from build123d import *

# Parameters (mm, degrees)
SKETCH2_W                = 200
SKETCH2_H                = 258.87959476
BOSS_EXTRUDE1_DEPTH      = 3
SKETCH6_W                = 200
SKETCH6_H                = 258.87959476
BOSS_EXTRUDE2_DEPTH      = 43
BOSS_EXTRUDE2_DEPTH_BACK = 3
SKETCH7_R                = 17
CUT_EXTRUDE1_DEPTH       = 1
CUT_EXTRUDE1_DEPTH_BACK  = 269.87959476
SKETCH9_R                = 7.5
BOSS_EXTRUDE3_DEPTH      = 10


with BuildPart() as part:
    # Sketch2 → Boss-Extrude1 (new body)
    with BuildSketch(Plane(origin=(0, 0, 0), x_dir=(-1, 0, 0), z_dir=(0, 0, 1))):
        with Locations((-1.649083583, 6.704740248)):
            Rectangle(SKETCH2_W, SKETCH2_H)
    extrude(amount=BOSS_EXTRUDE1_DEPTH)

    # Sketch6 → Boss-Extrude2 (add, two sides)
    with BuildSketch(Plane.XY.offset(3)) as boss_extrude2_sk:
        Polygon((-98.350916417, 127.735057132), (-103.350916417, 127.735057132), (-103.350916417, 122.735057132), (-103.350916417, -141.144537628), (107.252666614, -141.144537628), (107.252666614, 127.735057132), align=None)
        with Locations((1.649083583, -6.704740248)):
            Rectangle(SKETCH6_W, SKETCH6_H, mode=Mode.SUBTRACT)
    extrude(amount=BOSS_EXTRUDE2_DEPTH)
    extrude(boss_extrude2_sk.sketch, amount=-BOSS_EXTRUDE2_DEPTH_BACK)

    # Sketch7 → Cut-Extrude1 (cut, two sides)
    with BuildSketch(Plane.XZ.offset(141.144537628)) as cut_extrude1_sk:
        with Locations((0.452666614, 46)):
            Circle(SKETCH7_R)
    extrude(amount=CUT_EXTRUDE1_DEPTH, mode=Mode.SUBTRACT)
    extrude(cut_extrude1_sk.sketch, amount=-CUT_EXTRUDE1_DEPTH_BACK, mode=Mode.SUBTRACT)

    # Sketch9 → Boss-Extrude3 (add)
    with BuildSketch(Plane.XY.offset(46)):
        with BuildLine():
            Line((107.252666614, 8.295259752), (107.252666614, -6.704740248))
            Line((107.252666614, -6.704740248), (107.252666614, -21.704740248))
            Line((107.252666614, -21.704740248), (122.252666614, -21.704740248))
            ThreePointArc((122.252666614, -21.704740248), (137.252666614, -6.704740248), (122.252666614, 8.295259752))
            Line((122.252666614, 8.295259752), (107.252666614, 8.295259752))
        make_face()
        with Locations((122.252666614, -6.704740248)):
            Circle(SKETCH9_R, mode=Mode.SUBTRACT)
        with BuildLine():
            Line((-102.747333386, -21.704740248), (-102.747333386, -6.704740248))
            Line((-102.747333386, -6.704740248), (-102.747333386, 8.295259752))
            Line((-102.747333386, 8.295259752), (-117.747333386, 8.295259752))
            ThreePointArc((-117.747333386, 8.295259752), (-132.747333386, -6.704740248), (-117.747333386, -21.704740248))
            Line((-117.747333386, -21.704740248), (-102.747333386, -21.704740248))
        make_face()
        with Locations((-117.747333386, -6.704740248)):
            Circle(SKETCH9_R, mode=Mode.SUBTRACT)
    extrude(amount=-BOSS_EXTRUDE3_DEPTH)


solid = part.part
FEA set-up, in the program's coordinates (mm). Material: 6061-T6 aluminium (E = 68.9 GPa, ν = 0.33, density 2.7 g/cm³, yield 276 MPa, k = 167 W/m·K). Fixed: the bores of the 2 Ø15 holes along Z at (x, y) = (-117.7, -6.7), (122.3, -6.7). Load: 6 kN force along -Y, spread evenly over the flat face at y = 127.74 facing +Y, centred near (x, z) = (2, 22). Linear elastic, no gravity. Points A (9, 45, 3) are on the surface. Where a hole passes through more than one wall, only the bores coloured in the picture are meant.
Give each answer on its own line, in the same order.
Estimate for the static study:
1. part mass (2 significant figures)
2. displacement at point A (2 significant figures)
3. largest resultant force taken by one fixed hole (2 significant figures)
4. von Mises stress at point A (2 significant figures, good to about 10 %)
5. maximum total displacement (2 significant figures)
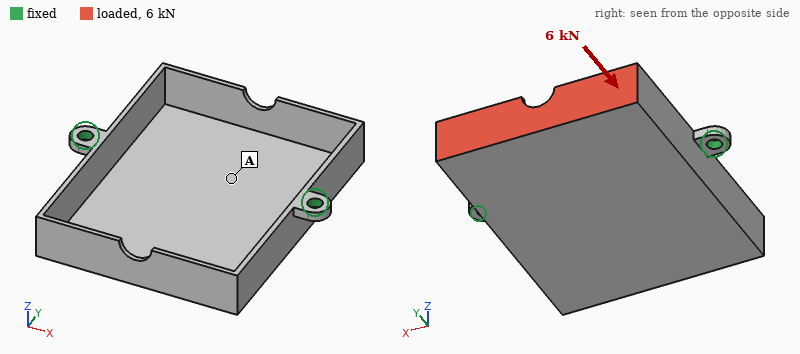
1.0 kg
0.55 mm
3.0 kN
18 MPa
1.4 mm
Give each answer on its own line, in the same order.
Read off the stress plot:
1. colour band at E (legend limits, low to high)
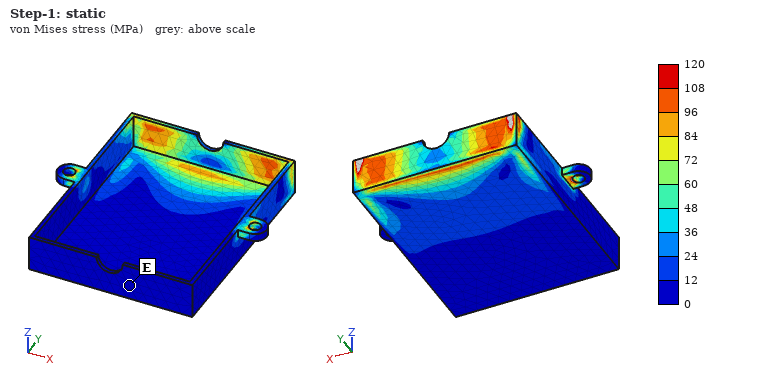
0 to 12 MPa
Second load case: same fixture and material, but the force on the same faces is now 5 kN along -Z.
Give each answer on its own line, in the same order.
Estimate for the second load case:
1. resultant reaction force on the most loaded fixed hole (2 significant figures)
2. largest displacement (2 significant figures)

2.5 kN
3.0 mm
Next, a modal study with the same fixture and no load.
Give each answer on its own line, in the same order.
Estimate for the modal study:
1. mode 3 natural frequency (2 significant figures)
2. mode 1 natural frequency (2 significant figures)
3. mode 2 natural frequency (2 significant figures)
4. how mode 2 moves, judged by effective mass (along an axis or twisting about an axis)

480 Hz
320 Hz
410 Hz
twisting about Z
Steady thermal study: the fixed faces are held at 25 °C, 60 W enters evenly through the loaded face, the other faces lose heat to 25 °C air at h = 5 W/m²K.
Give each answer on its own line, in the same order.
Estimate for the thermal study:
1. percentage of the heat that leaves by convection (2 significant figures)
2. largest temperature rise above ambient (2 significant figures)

34 %
58 K
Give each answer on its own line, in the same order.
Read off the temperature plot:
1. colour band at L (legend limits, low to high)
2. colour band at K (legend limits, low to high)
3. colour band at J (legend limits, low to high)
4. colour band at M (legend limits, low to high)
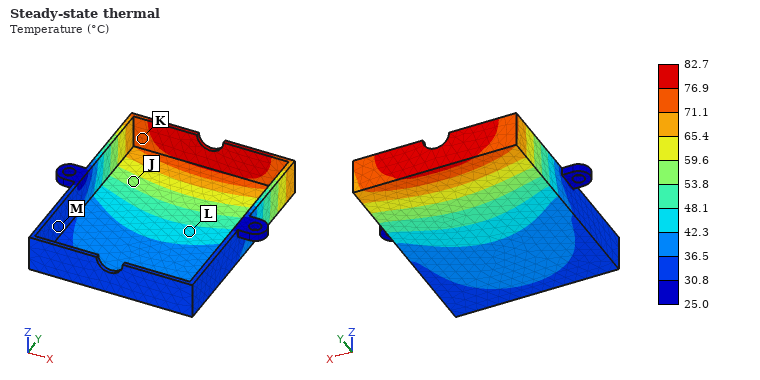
42.3 to 48.1 °C
71.1 to 76.9 °C
53.8 to 59.6 °C
30.8 to 36.5 °C
